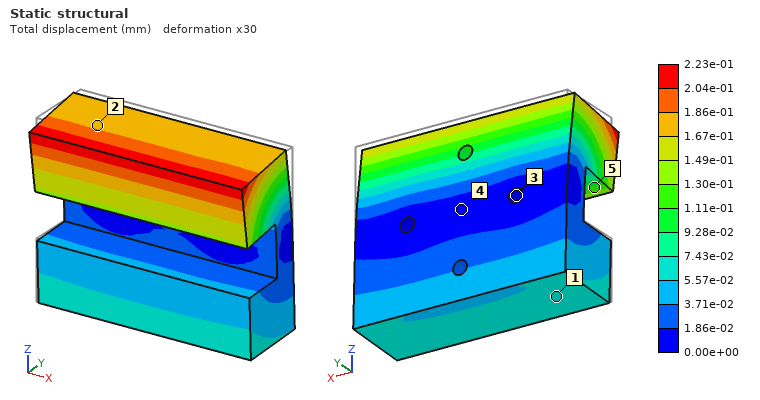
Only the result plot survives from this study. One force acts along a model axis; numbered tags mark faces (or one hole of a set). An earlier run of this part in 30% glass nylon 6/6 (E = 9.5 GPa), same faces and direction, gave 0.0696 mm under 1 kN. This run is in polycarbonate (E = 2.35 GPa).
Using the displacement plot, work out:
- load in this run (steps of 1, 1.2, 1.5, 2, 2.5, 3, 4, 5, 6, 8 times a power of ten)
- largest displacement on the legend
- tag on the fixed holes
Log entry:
800 N
2.23e-01 mm
3
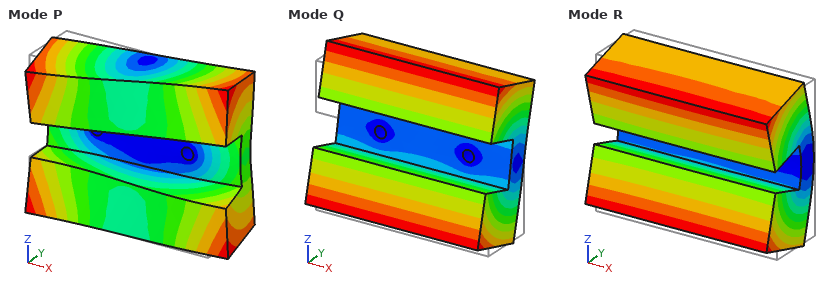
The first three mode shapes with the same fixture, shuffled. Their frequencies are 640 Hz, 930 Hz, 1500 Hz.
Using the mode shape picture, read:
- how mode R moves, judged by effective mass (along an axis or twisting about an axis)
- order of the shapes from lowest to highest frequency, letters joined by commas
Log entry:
along Y
Q, R, P
